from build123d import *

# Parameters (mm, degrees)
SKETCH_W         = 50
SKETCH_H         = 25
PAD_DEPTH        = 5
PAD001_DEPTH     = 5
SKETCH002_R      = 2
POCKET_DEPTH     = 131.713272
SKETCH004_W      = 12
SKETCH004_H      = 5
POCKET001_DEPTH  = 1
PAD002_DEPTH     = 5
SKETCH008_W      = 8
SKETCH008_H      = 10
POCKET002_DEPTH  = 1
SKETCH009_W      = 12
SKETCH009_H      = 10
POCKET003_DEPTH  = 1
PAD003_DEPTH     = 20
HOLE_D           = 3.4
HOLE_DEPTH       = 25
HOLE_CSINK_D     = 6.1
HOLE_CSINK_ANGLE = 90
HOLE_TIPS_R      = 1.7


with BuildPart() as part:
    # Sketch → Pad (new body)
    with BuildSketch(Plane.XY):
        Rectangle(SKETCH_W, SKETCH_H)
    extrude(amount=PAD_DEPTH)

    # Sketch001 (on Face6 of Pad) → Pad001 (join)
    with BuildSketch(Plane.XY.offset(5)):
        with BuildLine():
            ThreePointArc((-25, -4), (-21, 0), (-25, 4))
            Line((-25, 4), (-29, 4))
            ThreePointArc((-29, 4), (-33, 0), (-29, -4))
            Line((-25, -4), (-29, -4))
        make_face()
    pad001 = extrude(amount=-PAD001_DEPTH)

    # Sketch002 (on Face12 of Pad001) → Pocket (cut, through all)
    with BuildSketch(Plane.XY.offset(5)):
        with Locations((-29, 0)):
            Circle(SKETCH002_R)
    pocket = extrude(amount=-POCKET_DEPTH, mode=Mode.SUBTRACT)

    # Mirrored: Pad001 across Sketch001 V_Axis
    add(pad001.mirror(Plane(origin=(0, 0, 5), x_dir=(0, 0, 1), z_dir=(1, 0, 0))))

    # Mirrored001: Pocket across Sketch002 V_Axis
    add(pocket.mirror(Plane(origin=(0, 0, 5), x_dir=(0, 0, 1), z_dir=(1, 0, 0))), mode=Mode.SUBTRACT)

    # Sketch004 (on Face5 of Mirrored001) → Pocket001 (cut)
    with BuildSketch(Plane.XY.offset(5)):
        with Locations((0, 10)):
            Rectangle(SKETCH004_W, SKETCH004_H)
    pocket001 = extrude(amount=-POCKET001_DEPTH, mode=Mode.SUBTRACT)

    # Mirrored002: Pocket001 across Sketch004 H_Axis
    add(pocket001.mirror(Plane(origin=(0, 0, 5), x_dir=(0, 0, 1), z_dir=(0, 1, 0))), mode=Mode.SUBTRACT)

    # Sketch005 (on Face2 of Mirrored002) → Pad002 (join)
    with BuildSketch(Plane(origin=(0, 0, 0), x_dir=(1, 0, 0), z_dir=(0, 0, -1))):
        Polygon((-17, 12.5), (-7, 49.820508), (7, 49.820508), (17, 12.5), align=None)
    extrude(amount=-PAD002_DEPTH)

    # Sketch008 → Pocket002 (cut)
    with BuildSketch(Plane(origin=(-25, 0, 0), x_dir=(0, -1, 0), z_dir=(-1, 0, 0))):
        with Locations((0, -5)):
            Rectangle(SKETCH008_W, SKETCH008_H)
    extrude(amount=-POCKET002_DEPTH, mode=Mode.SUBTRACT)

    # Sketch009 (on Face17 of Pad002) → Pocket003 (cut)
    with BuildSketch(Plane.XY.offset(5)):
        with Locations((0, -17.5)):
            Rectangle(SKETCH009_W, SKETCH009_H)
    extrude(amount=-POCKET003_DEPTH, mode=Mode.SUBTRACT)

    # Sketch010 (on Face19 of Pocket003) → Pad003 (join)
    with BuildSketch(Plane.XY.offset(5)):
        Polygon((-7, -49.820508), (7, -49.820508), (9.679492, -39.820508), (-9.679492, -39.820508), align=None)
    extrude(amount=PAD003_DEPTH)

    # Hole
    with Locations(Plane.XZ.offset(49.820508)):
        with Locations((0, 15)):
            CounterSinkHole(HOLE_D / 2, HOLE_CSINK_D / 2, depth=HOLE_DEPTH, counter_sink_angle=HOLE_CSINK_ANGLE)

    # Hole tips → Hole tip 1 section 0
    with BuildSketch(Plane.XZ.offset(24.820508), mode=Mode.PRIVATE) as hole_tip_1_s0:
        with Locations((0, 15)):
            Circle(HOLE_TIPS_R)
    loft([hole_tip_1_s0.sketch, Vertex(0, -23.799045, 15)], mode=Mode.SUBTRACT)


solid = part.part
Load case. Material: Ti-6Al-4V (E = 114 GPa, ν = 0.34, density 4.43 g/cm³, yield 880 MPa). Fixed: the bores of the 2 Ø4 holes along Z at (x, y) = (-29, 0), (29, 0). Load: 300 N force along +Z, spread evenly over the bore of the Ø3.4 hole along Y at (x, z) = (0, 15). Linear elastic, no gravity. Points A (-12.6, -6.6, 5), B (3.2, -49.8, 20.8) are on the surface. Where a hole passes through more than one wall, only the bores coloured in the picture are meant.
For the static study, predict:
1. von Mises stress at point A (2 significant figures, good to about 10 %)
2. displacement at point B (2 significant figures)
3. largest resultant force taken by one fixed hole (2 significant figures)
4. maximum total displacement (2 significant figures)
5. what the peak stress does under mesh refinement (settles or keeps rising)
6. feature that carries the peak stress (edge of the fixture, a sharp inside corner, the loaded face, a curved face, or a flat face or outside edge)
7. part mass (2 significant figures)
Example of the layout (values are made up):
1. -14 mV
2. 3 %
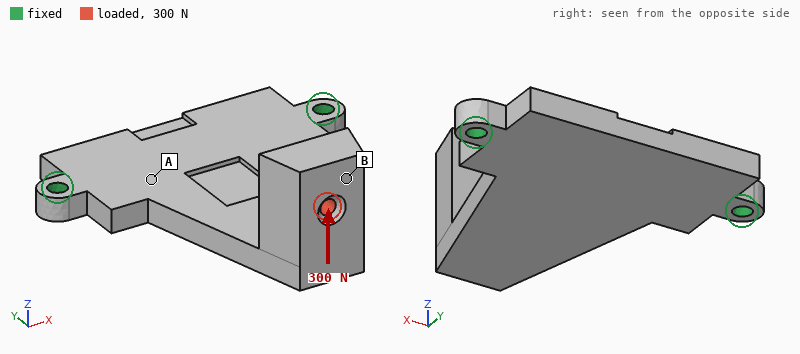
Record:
1. 72 MPa
2. 0.55 mm
3. 150 N
4. 0.58 mm
5. keeps rising
6. edge of the fixture
7. 63 g
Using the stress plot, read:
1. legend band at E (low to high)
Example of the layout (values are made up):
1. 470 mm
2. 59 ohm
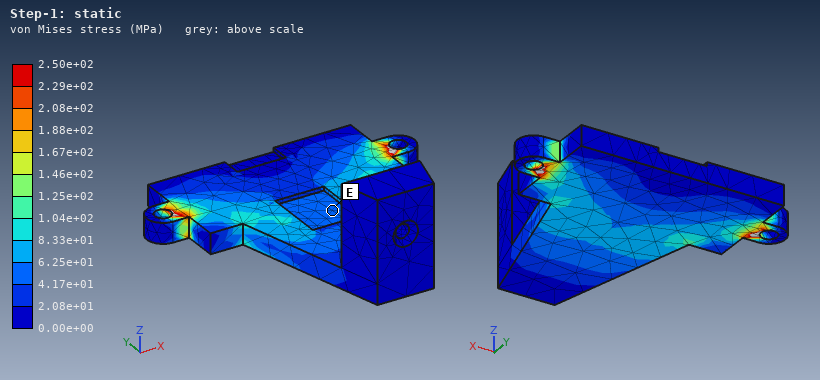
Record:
1. 4.17e+01 to 6.25e+01 MPa
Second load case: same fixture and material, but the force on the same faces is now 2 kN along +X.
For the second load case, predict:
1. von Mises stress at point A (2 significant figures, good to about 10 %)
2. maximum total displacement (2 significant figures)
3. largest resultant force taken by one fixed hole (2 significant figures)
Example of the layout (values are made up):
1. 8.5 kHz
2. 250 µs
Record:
1. 90 MPa
2. 0.54 mm
3. 2.0 kN
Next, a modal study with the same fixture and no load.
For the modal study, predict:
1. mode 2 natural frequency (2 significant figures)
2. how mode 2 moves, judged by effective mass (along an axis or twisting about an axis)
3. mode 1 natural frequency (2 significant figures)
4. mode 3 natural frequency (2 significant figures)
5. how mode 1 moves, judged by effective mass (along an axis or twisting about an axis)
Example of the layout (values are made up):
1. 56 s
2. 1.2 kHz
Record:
1. 2900 Hz
2. along X
3. 830 Hz
4. 3700 Hz
5. along Z
